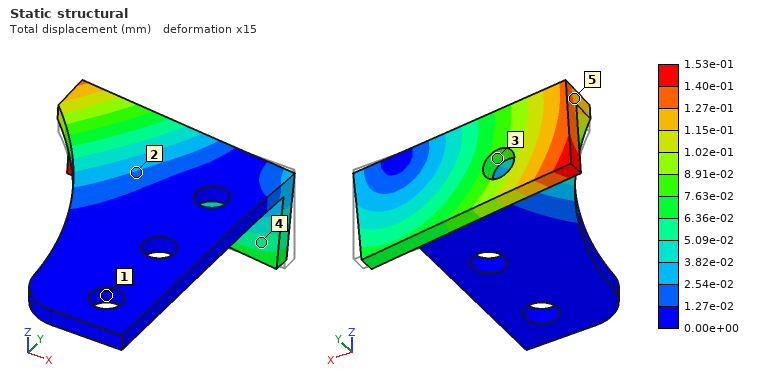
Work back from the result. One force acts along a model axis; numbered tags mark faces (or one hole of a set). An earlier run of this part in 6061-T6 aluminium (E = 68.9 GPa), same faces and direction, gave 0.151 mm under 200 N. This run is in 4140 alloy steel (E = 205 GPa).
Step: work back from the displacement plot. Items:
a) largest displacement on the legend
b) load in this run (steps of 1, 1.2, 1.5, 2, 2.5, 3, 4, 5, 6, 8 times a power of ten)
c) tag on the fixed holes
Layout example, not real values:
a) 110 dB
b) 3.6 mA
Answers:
a) 1.53e-01 mm
b) 600 N
c) 1
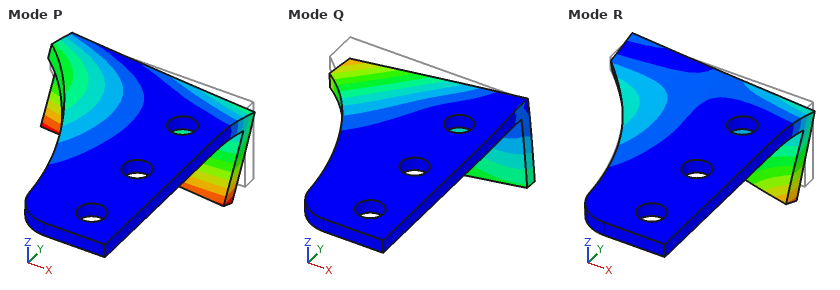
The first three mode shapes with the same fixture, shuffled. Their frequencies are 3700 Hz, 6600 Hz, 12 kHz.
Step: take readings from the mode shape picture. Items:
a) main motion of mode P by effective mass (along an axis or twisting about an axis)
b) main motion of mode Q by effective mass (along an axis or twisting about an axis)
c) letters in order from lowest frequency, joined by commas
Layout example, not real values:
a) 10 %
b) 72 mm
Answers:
a) along Y
b) along Z
c) Q, P, R
